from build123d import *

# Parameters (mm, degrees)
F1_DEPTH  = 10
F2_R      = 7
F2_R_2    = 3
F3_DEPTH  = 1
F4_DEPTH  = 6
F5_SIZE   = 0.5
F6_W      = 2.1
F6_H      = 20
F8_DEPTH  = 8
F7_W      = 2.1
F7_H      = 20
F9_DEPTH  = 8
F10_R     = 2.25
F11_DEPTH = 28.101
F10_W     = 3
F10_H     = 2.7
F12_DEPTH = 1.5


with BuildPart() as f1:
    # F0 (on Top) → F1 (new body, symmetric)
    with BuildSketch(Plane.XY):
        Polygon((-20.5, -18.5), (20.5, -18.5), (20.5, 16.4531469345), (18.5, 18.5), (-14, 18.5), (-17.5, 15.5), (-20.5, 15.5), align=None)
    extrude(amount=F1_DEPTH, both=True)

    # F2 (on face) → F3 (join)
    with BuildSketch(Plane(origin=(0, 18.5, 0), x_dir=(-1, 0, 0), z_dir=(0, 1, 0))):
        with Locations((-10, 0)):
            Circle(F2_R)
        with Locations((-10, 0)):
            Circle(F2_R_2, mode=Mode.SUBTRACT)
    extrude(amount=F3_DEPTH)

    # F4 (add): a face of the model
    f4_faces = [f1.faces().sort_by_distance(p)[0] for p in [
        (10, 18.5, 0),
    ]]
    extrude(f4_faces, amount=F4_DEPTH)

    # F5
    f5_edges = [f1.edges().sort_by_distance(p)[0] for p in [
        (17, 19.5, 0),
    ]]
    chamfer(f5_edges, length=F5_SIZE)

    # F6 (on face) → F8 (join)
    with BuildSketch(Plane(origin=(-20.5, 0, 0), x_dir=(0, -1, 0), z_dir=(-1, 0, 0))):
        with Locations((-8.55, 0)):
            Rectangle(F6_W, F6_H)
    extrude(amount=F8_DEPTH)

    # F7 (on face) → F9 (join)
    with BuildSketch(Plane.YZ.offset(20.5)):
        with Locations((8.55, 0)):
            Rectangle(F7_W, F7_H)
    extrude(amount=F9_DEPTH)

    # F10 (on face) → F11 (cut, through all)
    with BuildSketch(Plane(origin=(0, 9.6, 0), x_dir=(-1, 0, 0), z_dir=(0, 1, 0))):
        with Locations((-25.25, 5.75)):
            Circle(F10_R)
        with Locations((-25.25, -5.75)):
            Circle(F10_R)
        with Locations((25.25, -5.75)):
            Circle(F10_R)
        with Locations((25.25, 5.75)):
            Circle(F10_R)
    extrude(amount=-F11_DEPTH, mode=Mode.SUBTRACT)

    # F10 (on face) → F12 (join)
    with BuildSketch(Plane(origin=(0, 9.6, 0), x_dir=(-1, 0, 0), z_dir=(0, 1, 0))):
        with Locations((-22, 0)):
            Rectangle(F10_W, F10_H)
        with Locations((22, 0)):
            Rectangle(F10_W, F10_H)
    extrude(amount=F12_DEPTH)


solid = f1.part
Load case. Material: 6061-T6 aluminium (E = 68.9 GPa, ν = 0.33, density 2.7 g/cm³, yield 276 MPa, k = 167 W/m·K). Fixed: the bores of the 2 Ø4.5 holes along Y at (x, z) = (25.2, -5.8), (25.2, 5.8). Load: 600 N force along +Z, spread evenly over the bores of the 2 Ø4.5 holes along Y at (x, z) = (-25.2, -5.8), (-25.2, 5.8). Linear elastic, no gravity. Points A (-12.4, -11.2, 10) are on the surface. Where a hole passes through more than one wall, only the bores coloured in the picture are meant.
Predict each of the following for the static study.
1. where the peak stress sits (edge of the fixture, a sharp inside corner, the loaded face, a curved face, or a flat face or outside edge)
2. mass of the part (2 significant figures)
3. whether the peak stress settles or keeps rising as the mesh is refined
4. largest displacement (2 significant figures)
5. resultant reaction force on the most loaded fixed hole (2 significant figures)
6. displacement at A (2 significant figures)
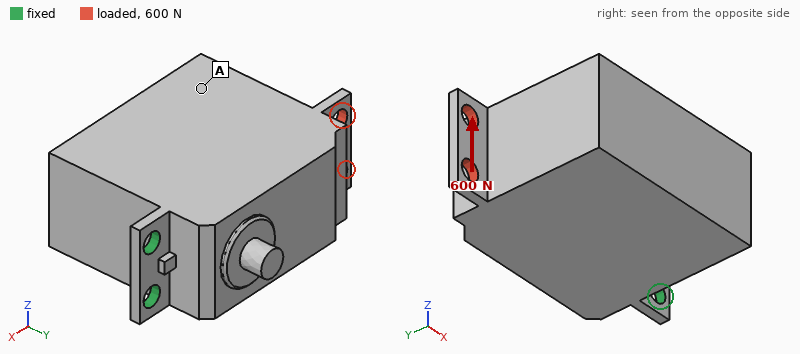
edge of the fixture
83 g
keeps rising
0.12 mm
2.2 kN
0.075 mm
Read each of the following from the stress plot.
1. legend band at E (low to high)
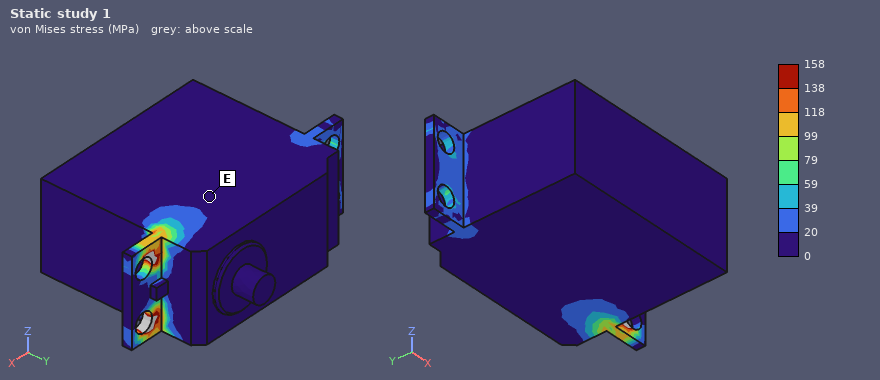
0 to 20 MPa
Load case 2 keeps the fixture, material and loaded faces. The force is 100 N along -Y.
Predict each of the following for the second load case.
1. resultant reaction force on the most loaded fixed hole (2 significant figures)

58 N
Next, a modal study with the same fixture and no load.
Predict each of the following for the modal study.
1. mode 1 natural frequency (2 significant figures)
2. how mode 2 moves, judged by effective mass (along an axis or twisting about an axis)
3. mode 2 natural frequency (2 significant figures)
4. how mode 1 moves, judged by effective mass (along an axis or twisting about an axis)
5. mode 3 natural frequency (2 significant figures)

370 Hz
along Z
2000 Hz
along Y
3400 Hz
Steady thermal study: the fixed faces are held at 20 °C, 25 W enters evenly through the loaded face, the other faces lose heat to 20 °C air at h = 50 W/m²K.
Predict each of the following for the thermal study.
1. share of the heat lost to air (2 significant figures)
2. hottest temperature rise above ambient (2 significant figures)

24 %
56 K
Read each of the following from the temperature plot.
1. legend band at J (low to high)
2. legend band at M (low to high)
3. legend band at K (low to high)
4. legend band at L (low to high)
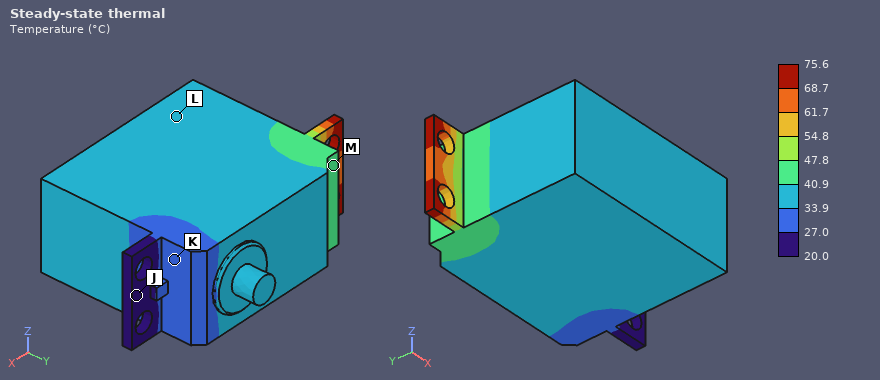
20.0 to 27.0 °C
40.9 to 47.8 °C
27.0 to 33.9 °C
33.9 to 40.9 °C
